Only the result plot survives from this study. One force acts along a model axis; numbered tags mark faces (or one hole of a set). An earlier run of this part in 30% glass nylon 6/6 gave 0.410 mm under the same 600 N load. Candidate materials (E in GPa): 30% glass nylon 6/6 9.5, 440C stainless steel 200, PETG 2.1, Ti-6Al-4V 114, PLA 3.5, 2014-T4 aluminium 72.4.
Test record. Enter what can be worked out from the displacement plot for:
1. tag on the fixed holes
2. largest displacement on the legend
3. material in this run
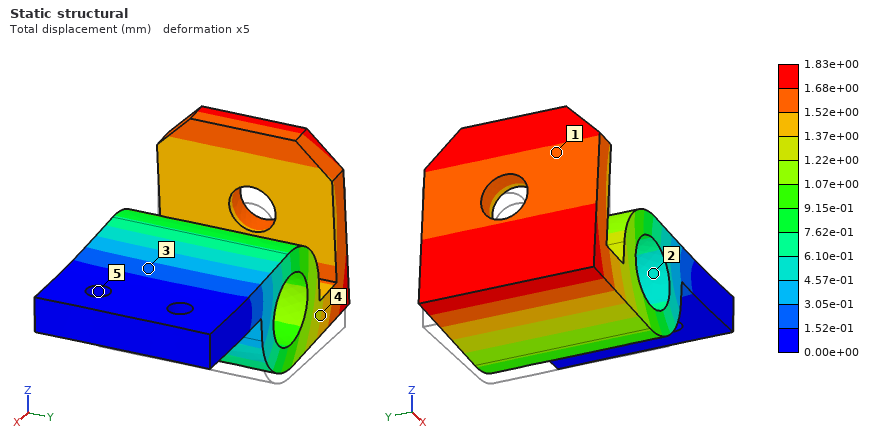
5
1.83e+00 mm
PETG
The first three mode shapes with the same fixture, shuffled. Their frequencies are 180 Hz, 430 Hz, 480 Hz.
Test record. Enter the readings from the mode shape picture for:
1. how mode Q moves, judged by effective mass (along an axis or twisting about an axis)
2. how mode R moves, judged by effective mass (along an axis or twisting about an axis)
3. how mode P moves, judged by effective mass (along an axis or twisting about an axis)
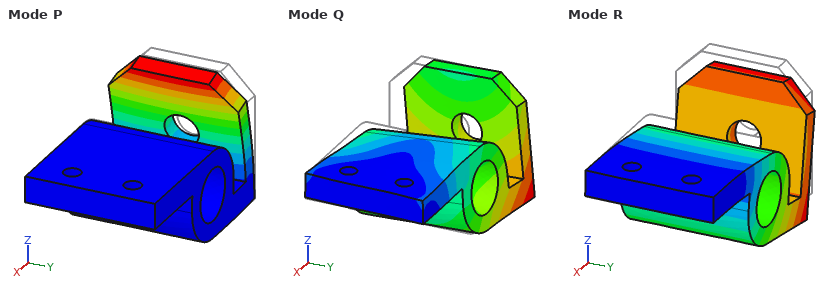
along Y
along Z
along X
